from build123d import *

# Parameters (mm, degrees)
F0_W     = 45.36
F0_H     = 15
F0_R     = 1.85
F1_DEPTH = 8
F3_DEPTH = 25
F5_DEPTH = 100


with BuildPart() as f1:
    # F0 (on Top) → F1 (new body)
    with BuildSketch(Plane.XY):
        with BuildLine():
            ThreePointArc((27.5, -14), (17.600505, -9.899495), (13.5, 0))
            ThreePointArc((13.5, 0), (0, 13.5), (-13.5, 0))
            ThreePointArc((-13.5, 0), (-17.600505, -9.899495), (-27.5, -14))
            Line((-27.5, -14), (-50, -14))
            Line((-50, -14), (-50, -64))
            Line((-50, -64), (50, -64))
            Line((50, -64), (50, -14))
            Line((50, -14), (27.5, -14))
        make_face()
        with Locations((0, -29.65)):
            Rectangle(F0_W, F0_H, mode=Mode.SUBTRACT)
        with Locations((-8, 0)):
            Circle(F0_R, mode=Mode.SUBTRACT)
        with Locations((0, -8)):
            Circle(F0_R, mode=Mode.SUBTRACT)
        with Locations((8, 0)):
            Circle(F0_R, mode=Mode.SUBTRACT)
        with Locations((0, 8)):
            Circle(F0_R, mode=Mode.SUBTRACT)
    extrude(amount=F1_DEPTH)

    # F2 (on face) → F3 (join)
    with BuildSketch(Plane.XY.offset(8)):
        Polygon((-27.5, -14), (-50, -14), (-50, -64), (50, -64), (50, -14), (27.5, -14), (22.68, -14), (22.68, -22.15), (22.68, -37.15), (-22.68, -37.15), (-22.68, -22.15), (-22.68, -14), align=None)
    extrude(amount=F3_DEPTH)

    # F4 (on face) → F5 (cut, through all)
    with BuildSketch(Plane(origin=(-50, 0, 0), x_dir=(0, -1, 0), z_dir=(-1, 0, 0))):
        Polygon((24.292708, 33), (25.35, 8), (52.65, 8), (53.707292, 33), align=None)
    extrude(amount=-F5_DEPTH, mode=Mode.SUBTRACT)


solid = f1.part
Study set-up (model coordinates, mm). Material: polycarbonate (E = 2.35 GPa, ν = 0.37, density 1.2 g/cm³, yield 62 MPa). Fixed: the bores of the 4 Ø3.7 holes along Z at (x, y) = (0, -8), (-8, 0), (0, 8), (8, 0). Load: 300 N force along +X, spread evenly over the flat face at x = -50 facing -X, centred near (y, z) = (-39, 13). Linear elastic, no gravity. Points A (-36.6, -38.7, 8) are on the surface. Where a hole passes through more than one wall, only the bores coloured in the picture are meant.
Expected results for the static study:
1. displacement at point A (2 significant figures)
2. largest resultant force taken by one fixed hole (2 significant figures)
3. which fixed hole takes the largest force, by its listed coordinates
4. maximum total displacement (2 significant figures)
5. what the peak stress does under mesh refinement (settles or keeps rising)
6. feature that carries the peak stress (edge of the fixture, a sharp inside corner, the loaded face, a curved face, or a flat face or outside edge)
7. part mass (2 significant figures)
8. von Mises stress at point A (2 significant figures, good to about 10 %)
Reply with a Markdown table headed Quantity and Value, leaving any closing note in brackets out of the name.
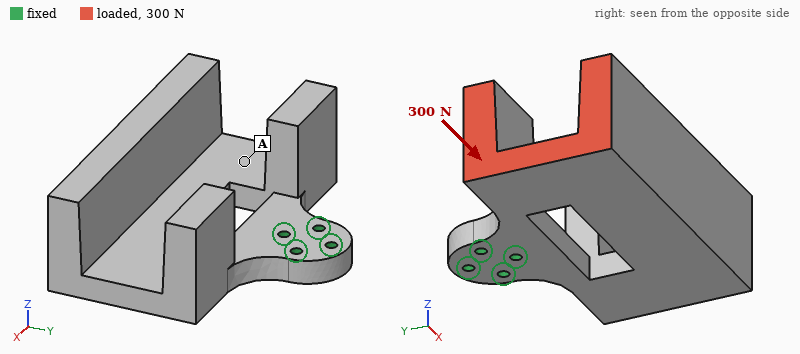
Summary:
| Quantity | Value |
|---|---|
| displacement at point A | 0.79 mm |
| largest resultant force taken by one fixed hole | 530 N |
| which fixed hole takes the largest force, by its listed coordinates | (0, -8) |
| maximum total displacement | 1.4 mm |
| what the peak stress does under mesh refinement | keeps rising |
| feature that carries the peak stress | edge of the fixture |
| part mass | 98 g |
| von Mises stress at point A | 2.3 MPa |
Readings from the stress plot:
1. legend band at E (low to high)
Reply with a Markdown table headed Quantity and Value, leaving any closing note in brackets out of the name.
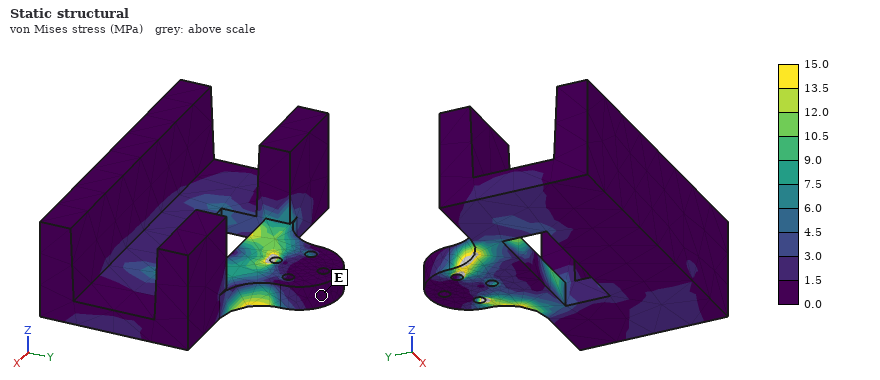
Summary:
| Quantity | Value |
|---|---|
| legend band at E | 0.0 to 1.5 MPa |
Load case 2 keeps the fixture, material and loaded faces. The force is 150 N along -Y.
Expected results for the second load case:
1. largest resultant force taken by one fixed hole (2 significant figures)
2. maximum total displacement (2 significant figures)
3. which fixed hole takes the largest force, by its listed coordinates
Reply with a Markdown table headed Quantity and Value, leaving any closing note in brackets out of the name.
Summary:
| Quantity | Value |
|---|---|
| largest resultant force taken by one fixed hole | 370 N |
| maximum total displacement | 1.4 mm |
| which fixed hole takes the largest force, by its listed coordinates | (-8, 0) |
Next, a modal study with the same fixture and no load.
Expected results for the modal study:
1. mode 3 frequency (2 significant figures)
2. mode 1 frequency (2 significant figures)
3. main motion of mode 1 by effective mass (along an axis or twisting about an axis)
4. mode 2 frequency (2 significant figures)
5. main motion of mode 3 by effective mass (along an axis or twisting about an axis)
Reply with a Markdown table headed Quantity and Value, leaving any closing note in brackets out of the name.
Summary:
| Quantity | Value |
|---|---|
| mode 3 frequency | 350 Hz |
| mode 1 frequency | 130 Hz |
| main motion of mode 1 by effective mass | along Z |
| mode 2 frequency | 210 Hz |
| main motion of mode 3 by effective mass | along X |
